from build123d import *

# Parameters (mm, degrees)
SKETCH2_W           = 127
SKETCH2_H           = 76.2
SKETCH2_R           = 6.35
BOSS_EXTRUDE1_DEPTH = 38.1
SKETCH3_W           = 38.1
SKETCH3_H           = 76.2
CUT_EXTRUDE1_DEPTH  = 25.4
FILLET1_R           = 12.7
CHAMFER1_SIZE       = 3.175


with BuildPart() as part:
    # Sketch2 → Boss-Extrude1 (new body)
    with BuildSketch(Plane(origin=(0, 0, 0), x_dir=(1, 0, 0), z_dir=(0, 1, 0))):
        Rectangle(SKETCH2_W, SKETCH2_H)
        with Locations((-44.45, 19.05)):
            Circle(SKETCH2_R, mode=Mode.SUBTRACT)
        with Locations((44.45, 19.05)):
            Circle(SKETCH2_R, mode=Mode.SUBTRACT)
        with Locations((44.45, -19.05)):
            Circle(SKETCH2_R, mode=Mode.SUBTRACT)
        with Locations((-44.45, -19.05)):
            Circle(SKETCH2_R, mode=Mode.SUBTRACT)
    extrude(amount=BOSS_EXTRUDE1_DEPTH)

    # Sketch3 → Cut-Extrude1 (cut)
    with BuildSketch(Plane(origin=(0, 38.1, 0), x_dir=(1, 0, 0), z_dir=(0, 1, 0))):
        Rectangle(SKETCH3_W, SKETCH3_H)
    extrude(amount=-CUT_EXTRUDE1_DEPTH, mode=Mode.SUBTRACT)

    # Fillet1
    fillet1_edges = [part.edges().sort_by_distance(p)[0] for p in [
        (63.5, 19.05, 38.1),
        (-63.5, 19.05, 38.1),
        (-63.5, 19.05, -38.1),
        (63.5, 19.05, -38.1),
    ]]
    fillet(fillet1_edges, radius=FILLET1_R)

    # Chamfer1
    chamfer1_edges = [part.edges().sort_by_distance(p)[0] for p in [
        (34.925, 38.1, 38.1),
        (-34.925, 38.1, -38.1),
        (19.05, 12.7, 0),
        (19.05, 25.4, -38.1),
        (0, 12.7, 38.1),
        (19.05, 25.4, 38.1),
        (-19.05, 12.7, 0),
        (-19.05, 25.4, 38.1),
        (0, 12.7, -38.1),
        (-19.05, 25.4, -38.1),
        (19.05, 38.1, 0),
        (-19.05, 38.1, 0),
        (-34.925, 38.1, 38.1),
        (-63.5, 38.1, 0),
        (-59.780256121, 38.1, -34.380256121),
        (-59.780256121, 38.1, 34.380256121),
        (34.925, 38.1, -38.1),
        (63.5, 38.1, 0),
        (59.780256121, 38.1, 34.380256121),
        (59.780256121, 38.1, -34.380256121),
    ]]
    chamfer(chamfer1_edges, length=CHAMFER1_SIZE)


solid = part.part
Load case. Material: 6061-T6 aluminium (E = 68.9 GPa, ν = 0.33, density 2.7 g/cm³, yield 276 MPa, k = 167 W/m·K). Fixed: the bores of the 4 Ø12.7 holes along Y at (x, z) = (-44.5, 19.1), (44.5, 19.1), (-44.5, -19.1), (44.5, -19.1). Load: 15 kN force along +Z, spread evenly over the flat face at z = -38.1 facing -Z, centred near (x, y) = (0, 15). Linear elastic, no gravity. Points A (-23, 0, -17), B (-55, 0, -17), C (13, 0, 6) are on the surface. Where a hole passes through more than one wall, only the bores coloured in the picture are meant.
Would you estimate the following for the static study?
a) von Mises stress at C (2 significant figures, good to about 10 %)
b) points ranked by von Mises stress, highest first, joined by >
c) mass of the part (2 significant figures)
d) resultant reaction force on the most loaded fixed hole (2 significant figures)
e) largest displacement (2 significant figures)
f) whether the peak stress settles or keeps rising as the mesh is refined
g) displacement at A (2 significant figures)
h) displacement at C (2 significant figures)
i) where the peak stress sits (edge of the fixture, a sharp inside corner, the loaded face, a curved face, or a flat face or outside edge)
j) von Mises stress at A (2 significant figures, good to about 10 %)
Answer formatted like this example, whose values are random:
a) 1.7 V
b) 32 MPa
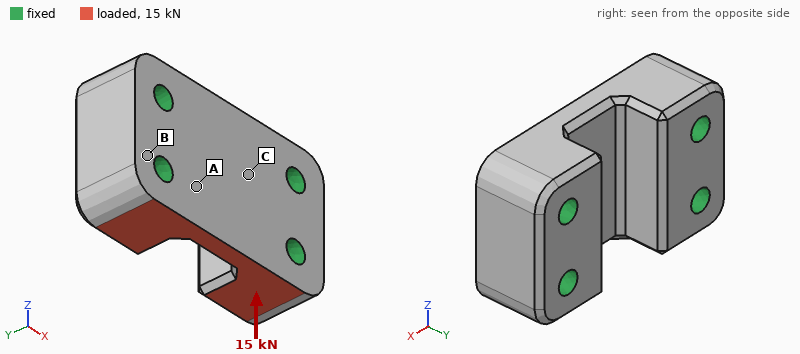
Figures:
a) 2.9 MPa
b) A > C > B
c) 720 g
d) 5.9 kN
e) 5.8 µm
f) keeps rising
g) 2.4 µm
h) 1.9 µm
i) edge of the fixture
j) 5.2 MPa
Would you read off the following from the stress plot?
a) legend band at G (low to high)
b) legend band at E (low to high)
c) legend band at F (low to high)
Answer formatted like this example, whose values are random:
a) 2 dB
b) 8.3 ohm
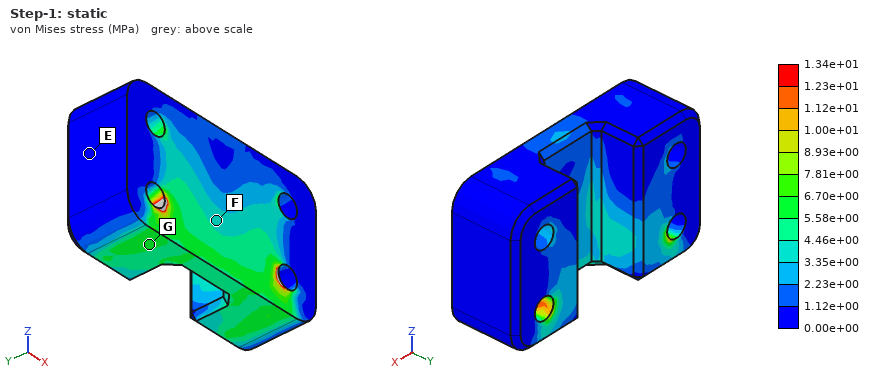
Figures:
a) 5.58e+00 to 6.70e+00 MPa
b) 0.00e+00 to 1.12e+00 MPa
c) 3.35e+00 to 4.46e+00 MPa
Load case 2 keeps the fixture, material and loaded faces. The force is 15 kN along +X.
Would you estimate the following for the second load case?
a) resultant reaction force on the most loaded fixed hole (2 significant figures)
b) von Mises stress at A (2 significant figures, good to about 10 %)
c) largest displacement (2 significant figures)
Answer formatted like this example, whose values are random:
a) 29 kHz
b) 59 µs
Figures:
a) 8.0 kN
b) 4.9 MPa
c) 5.7 µm
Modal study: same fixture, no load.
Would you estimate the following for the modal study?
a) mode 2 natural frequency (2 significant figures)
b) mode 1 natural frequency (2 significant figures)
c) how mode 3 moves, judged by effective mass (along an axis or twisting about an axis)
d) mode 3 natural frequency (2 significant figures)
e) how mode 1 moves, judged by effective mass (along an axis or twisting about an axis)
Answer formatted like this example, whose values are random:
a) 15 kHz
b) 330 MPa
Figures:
a) 17 kHz
b) 17 kHz
c) along Z
d) 20 kHz
e) along Y
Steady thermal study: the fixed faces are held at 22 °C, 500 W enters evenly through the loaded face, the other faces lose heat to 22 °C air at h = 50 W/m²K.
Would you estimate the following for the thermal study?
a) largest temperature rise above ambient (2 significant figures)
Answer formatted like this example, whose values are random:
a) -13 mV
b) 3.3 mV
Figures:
a) 30 K
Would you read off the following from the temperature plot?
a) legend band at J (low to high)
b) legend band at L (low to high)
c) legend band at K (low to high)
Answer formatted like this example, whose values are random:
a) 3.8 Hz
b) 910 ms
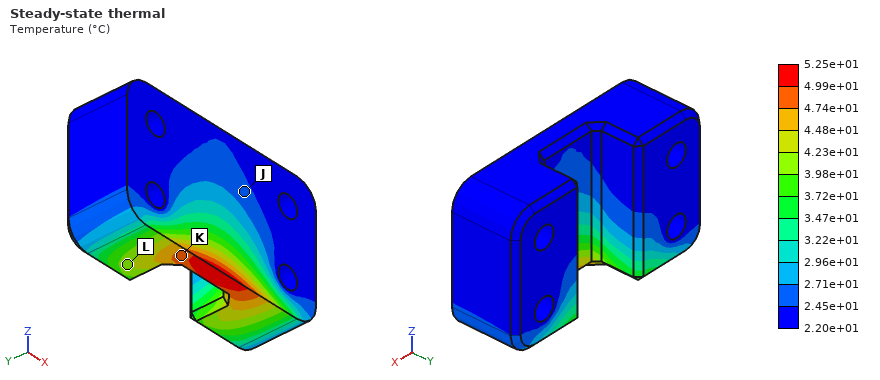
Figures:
a) 2.45e+01 to 2.71e+01 °C
b) 3.98e+01 to 4.23e+01 °C
c) 4.74e+01 to 4.99e+01 °C
